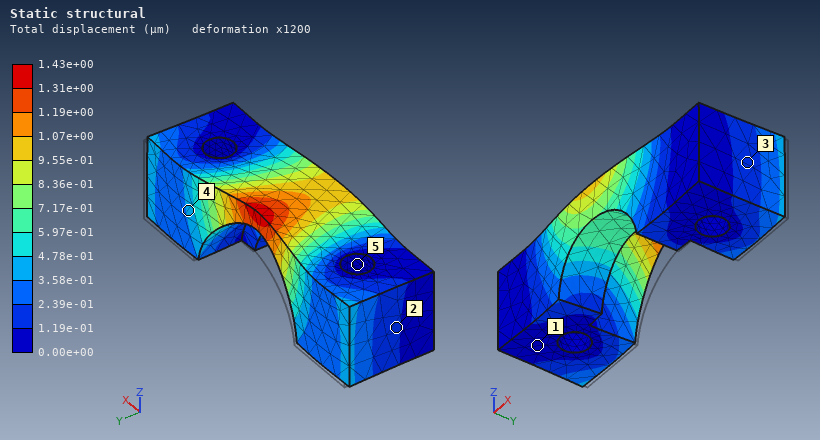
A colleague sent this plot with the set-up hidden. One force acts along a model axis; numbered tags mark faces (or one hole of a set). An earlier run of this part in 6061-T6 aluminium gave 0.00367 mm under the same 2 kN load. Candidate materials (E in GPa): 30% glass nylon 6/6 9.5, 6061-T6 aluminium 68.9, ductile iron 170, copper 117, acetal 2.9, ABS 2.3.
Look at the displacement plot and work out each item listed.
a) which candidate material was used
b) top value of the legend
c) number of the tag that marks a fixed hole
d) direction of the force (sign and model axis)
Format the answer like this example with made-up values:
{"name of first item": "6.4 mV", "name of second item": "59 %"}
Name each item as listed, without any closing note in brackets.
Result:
{"which candidate material was used": "ductile iron", "top value of the legend": "1.43e+00 µm", "number of the tag that marks a fixed hole": "5", "direction of the force": "-Y"}
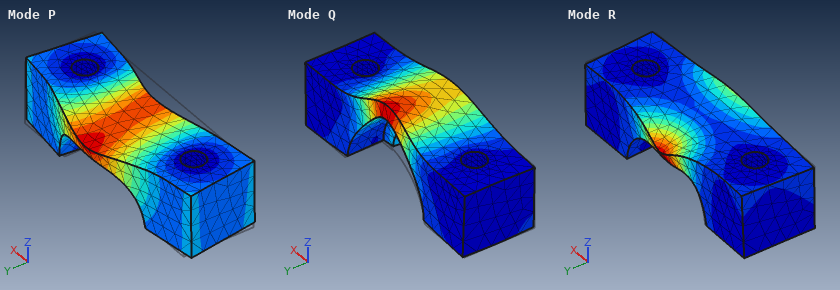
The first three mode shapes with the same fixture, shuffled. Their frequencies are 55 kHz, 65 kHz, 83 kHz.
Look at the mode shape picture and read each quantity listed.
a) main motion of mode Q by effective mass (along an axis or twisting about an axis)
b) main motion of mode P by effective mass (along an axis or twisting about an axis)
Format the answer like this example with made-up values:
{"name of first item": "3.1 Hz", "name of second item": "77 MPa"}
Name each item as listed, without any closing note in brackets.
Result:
{"main motion of mode Q by effective mass": "along Z", "main motion of mode P by effective mass": "along Y"}
